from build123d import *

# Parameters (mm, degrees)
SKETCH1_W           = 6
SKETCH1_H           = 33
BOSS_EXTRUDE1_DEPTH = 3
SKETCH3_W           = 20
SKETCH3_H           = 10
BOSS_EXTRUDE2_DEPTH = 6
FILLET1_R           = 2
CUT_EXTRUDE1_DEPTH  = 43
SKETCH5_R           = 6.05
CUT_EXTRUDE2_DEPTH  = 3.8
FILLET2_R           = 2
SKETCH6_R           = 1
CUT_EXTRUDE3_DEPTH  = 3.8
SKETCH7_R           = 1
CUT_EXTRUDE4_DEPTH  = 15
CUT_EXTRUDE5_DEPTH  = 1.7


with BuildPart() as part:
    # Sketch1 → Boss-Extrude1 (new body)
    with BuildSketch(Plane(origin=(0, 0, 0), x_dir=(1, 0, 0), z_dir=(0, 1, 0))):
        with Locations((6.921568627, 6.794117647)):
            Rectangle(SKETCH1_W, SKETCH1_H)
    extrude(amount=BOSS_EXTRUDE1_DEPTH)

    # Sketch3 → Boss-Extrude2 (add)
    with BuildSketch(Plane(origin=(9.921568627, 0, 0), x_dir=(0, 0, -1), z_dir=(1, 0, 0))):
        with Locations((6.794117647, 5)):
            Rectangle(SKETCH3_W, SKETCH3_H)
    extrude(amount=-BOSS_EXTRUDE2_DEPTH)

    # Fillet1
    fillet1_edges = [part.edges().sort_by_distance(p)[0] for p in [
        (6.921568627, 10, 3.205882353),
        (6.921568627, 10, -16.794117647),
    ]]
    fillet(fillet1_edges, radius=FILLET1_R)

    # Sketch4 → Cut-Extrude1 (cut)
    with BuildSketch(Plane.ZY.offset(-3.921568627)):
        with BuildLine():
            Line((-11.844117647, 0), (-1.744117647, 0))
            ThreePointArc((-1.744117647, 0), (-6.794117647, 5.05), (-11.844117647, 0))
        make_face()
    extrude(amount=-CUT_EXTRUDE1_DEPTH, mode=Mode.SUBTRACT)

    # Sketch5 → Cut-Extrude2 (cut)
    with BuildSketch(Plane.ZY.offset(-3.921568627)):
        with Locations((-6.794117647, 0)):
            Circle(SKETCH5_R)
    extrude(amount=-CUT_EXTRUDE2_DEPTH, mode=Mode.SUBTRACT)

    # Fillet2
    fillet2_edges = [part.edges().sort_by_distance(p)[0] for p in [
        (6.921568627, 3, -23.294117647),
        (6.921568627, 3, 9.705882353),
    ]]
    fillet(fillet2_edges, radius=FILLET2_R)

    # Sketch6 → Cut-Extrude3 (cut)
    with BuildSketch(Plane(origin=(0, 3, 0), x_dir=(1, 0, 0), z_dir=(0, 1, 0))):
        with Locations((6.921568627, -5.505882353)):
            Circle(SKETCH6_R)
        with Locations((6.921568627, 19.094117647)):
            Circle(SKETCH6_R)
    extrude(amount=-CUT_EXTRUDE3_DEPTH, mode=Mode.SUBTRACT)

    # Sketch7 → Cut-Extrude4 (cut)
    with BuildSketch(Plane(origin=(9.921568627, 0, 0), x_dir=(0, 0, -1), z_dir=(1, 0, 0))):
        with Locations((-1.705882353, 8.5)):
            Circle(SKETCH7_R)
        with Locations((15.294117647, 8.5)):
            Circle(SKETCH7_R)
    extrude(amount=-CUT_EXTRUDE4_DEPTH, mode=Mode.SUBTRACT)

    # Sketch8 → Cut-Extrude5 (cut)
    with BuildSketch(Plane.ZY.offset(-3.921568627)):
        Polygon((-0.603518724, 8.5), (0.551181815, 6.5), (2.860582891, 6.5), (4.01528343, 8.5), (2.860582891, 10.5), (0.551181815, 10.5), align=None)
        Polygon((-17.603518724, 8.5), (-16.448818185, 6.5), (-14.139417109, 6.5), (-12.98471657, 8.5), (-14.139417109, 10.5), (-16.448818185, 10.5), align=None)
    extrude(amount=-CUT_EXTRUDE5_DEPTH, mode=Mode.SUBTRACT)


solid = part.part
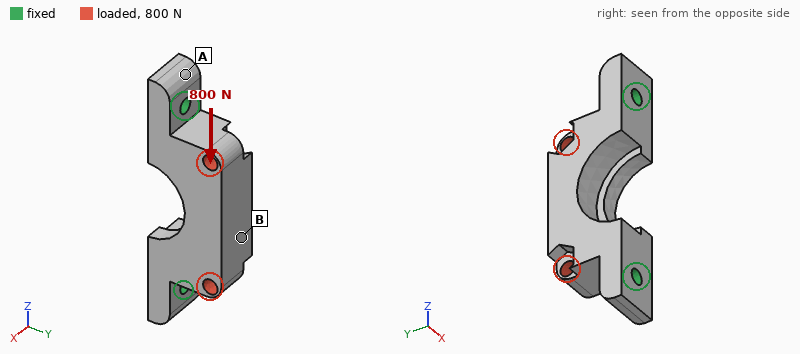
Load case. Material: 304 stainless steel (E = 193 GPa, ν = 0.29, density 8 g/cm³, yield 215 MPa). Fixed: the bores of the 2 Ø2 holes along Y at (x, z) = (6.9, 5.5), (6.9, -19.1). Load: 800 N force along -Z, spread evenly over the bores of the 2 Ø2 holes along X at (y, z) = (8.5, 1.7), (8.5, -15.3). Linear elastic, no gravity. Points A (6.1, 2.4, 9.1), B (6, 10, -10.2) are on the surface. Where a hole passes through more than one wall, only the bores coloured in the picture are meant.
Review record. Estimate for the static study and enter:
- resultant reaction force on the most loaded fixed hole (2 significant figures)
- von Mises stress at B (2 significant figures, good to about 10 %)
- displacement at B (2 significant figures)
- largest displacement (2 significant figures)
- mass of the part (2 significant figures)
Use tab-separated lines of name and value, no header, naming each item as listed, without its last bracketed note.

resultant reaction force on the most loaded fixed hole	470 N
von Mises stress at B	26 MPa
displacement at B	2.1 µm
largest displacement	4.2 µm
mass of the part	8.2 g
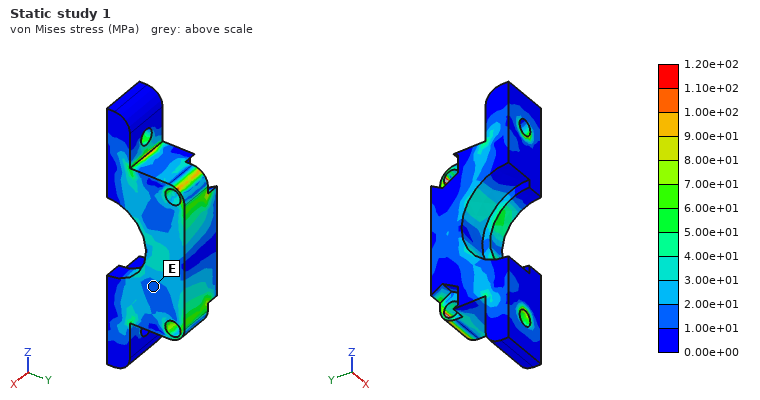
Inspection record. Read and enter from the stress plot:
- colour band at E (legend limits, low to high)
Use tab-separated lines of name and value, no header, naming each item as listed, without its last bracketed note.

colour band at E	1.00e+01 to 2.00e+01 MPa
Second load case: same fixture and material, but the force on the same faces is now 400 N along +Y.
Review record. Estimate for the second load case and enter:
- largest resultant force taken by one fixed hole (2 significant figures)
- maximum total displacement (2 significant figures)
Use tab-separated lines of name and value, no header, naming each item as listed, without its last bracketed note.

largest resultant force taken by one fixed hole	210 N
maximum total displacement	2.8 µm
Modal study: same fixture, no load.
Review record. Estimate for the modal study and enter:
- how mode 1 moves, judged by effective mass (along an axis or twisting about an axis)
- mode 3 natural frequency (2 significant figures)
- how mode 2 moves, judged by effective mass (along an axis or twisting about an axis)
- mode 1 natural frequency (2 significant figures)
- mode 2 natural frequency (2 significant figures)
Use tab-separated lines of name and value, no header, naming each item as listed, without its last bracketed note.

how mode 1 moves, judged by effective mass	along X
mode 3 natural frequency	41 kHz
how mode 2 moves, judged by effective mass	along Y
mode 1 natural frequency	14 kHz
mode 2 natural frequency	37 kHz
